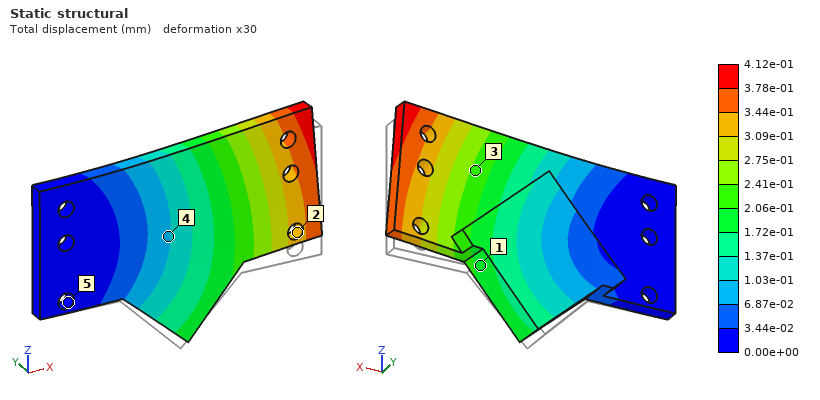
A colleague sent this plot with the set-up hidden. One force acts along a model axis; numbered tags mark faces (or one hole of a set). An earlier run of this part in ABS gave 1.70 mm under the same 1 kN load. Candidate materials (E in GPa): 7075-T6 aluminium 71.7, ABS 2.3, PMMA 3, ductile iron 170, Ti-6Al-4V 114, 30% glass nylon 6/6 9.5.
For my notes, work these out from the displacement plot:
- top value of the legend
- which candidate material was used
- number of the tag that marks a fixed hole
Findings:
4.12e-01 mm
30% glass nylon 6/6
5
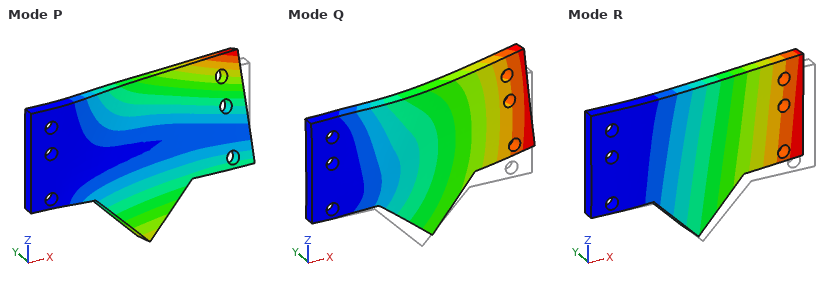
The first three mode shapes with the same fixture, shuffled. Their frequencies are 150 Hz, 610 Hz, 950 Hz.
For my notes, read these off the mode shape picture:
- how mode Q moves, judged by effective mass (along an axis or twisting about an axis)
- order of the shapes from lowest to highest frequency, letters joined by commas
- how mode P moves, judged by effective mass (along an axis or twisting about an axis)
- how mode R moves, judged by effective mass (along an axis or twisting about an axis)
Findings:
along Z
R, P, Q
twisting about X
along Y
